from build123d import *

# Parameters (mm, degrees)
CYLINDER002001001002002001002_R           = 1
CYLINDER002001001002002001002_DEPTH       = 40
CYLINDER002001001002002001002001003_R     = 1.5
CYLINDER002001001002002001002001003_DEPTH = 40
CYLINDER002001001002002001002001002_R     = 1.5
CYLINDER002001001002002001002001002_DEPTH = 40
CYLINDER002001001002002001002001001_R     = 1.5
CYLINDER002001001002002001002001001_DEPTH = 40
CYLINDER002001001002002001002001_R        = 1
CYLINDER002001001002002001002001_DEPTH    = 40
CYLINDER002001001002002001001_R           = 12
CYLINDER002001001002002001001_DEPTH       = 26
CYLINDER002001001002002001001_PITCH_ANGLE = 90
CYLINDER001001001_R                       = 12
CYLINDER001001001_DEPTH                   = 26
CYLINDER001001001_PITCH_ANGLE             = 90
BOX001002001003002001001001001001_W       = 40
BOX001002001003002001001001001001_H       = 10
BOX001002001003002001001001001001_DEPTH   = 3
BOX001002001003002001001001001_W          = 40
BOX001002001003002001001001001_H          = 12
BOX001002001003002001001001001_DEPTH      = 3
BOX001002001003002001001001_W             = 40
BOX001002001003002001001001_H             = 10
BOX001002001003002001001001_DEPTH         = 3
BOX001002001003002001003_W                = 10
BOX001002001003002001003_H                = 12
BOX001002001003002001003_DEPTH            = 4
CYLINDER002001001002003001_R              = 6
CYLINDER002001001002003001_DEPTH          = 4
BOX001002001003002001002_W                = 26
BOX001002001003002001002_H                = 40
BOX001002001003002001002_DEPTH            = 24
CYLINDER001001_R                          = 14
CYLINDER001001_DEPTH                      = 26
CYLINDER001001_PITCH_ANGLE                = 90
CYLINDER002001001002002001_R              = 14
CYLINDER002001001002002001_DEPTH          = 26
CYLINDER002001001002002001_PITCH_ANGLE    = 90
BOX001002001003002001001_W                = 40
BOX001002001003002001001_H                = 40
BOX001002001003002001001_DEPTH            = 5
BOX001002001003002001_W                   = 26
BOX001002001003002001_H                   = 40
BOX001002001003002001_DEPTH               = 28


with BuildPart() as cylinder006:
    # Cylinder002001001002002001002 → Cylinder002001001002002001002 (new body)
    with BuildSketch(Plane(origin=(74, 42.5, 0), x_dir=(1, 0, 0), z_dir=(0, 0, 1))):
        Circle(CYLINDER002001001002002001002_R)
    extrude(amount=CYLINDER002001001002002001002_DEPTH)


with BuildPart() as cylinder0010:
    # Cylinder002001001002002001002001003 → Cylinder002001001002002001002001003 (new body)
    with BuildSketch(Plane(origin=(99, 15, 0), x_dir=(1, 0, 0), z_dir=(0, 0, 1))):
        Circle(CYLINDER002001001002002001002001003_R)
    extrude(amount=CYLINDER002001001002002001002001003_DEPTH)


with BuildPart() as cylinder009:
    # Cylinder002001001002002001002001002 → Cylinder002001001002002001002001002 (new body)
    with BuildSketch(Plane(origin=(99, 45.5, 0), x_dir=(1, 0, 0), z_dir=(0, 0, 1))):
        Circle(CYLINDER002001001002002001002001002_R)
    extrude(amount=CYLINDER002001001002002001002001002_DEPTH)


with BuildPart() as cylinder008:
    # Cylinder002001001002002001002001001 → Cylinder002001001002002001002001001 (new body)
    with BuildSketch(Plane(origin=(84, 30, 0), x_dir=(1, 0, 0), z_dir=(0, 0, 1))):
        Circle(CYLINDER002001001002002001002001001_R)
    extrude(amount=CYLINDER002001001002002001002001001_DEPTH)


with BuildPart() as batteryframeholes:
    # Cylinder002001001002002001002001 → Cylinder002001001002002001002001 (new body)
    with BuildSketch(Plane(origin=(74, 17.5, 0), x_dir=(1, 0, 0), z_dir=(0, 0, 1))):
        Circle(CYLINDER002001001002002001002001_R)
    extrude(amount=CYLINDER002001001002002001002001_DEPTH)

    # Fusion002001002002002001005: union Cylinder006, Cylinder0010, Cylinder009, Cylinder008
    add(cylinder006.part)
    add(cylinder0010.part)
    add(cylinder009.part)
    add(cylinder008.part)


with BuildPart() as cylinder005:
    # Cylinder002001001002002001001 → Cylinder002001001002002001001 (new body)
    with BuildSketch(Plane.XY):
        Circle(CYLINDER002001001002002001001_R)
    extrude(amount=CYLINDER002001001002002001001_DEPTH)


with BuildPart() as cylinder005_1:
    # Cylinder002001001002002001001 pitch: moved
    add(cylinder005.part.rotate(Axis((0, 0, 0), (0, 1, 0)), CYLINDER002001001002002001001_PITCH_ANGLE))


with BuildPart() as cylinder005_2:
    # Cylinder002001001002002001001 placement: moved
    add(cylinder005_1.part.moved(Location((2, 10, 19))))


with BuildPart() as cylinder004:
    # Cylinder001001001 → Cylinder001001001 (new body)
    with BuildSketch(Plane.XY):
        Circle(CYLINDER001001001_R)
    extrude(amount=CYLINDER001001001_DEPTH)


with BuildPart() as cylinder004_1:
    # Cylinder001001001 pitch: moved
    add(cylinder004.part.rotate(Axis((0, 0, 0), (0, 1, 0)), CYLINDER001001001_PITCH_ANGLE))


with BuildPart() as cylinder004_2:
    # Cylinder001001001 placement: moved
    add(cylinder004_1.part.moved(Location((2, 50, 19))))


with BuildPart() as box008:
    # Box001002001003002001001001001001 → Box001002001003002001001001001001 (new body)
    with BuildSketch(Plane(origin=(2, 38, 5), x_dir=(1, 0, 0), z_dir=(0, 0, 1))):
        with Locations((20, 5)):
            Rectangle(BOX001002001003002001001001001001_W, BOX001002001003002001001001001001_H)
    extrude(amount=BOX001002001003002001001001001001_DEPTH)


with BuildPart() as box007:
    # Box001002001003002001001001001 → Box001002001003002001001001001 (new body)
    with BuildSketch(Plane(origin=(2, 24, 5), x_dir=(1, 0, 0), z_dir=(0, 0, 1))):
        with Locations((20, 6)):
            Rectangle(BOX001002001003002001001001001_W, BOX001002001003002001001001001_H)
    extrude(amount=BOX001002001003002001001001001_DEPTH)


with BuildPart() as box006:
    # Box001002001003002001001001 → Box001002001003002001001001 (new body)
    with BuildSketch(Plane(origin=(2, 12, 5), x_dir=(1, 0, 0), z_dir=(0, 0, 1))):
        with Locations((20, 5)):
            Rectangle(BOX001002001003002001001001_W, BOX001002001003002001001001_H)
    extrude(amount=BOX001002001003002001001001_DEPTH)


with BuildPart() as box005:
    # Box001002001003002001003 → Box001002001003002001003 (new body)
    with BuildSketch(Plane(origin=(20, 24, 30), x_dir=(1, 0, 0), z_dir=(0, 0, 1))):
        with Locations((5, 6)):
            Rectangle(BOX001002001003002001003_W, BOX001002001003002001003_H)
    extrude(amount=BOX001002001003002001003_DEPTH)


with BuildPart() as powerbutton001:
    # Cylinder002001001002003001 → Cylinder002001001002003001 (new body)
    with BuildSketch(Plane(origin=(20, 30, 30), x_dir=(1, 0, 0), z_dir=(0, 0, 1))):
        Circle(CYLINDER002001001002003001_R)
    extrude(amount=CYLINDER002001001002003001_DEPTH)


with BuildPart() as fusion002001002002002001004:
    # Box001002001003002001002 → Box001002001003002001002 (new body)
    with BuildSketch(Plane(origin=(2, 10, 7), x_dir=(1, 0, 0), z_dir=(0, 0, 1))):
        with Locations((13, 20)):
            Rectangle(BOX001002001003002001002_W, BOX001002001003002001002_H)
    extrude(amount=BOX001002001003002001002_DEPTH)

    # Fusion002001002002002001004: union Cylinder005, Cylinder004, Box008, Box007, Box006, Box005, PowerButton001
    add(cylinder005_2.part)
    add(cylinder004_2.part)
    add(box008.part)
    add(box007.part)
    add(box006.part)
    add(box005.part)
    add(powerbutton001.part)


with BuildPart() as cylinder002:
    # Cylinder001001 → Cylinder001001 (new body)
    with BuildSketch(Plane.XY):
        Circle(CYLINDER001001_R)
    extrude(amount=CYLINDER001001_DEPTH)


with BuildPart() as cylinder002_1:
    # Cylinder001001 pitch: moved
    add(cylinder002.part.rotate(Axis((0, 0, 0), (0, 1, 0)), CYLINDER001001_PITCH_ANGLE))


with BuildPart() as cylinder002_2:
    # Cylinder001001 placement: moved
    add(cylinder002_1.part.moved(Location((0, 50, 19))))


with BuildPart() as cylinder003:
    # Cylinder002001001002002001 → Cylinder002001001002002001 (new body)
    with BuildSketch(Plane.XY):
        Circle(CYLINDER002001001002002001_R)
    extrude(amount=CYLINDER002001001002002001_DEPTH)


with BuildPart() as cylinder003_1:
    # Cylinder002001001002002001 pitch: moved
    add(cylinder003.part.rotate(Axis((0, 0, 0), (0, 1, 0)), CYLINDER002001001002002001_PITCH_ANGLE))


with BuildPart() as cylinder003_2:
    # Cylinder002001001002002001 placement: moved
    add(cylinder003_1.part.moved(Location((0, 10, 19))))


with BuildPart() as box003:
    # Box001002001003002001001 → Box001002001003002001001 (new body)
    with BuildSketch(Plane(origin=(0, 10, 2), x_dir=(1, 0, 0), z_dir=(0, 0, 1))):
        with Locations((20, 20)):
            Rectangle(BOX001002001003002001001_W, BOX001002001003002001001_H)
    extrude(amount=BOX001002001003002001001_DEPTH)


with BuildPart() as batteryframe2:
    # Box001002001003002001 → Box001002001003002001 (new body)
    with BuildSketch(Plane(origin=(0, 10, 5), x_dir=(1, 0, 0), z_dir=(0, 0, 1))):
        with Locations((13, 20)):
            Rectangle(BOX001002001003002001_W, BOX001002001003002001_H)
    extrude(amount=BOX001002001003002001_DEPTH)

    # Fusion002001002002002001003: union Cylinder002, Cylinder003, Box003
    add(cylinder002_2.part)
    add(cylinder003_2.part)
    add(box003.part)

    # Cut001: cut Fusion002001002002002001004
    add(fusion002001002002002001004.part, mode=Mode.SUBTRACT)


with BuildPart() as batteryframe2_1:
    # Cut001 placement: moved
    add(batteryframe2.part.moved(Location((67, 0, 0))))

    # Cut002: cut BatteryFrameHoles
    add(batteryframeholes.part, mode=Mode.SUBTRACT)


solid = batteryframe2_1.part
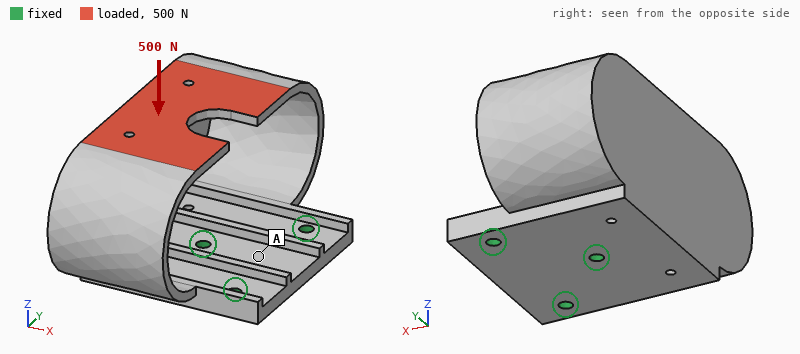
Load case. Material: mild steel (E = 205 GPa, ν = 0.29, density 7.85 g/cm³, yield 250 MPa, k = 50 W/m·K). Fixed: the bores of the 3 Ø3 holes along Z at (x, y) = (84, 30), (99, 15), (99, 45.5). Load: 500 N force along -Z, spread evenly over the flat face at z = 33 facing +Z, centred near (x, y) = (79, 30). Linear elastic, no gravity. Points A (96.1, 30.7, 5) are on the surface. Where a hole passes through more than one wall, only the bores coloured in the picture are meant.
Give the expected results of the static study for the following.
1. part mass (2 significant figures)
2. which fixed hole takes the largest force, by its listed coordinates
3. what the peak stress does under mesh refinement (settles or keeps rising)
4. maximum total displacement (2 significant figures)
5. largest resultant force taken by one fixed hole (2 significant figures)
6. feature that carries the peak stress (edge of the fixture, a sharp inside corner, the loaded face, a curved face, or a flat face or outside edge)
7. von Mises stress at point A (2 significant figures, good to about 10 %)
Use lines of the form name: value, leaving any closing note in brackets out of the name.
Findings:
part mass: 110 g
which fixed hole takes the largest force, by its listed coordinates: (84, 30)
what the peak stress does under mesh refinement: keeps rising
maximum total displacement: 0.14 mm
largest resultant force taken by one fixed hole: 400 N
feature that carries the peak stress: edge of the fixture
von Mises stress at point A: 9.0 MPa
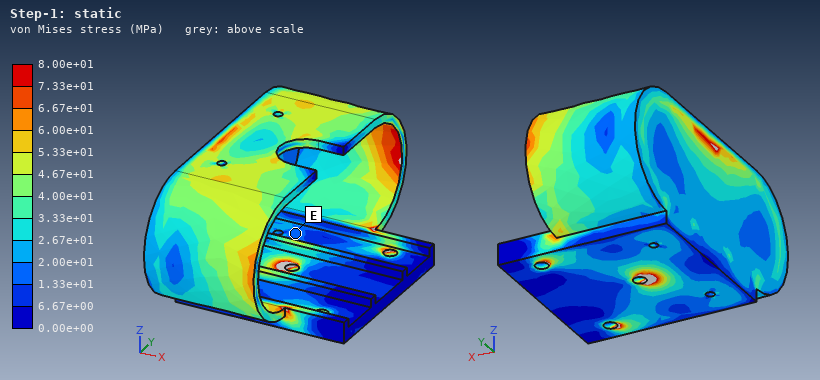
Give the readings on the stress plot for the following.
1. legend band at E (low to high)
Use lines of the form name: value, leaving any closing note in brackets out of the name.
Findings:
legend band at E: 1.33e+01 to 2.00e+01 MPa
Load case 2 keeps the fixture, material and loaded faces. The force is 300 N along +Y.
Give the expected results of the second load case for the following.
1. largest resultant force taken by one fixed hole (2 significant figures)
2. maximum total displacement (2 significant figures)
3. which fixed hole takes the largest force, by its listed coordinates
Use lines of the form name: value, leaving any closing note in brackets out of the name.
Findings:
largest resultant force taken by one fixed hole: 260 N
maximum total displacement: 0.14 mm
which fixed hole takes the largest force, by its listed coordinates: (84, 30)
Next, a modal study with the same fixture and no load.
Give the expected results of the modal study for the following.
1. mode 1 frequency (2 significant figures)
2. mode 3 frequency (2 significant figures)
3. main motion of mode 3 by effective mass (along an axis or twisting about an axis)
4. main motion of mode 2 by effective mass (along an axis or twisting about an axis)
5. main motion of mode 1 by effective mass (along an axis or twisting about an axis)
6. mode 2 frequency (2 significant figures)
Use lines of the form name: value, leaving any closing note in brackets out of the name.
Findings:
mode 1 frequency: 1100 Hz
mode 3 frequency: 2500 Hz
main motion of mode 3 by effective mass: along Z
main motion of mode 2 by effective mass: along X
main motion of mode 1 by effective mass: along Y
mode 2 frequency: 1600 Hz
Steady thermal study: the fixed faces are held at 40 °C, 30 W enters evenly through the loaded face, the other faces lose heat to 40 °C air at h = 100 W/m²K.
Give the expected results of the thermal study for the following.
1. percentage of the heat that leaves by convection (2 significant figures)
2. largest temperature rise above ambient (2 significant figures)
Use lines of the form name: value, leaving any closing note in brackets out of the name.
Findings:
percentage of the heat that leaves by convection: 87 %
largest temperature rise above ambient: 74 K
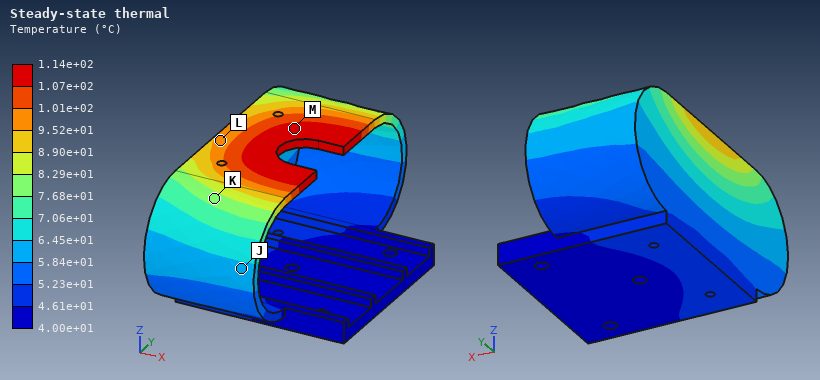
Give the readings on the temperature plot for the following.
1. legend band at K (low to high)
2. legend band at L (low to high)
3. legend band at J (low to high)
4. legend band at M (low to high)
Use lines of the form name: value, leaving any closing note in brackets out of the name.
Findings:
legend band at K: 7.68e+01 to 8.29e+01 °C
legend band at L: 9.52e+01 to 1.01e+02 °C
legend band at J: 5.84e+01 to 6.45e+01 °C
legend band at M: 1.07e+02 to 1.14e+02 °C
